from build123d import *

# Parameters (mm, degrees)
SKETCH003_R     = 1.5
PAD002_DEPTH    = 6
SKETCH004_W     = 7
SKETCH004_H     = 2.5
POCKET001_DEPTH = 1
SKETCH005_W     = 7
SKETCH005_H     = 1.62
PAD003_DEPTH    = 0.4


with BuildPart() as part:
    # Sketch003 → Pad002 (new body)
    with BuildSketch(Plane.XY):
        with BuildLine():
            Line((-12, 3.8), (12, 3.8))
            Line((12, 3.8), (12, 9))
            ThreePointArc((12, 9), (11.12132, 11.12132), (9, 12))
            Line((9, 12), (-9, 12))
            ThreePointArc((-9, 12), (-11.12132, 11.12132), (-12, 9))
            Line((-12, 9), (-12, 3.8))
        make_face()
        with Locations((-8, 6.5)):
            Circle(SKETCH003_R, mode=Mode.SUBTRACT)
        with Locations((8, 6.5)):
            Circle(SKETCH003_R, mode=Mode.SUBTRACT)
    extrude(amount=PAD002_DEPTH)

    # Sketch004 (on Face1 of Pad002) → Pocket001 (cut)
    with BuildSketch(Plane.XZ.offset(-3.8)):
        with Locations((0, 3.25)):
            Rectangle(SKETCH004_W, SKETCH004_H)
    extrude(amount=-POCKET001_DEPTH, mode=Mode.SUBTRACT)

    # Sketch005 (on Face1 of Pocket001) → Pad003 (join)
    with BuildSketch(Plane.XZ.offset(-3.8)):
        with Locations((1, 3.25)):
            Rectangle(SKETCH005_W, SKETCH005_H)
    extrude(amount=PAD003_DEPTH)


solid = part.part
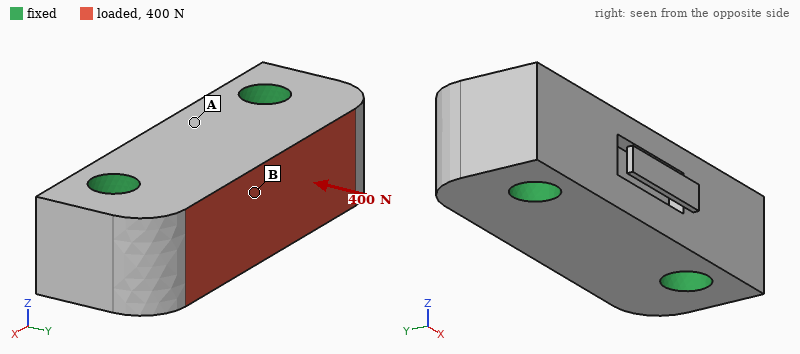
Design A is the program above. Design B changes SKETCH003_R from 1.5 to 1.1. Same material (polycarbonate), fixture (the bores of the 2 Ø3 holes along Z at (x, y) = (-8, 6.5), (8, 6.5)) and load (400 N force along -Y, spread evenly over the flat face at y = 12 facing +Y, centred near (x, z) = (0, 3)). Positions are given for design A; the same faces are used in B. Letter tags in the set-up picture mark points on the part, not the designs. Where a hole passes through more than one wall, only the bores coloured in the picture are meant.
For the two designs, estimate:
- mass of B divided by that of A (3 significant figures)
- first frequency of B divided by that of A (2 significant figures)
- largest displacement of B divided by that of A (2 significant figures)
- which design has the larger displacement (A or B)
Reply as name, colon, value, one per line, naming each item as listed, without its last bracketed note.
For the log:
mass of B divided by that of A: 1.04
first frequency of B divided by that of A: 1.0
largest displacement of B divided by that of A: 1.3
which design has the larger displacement: B
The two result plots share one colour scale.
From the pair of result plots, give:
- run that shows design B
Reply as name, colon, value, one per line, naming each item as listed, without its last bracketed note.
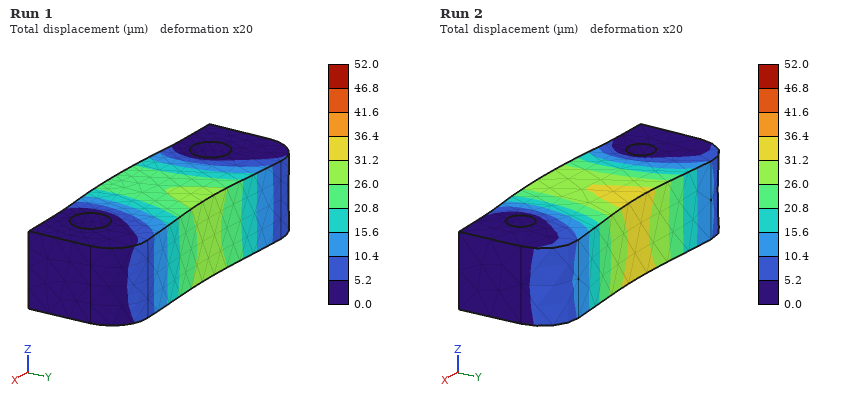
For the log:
run that shows design B: Run 2
